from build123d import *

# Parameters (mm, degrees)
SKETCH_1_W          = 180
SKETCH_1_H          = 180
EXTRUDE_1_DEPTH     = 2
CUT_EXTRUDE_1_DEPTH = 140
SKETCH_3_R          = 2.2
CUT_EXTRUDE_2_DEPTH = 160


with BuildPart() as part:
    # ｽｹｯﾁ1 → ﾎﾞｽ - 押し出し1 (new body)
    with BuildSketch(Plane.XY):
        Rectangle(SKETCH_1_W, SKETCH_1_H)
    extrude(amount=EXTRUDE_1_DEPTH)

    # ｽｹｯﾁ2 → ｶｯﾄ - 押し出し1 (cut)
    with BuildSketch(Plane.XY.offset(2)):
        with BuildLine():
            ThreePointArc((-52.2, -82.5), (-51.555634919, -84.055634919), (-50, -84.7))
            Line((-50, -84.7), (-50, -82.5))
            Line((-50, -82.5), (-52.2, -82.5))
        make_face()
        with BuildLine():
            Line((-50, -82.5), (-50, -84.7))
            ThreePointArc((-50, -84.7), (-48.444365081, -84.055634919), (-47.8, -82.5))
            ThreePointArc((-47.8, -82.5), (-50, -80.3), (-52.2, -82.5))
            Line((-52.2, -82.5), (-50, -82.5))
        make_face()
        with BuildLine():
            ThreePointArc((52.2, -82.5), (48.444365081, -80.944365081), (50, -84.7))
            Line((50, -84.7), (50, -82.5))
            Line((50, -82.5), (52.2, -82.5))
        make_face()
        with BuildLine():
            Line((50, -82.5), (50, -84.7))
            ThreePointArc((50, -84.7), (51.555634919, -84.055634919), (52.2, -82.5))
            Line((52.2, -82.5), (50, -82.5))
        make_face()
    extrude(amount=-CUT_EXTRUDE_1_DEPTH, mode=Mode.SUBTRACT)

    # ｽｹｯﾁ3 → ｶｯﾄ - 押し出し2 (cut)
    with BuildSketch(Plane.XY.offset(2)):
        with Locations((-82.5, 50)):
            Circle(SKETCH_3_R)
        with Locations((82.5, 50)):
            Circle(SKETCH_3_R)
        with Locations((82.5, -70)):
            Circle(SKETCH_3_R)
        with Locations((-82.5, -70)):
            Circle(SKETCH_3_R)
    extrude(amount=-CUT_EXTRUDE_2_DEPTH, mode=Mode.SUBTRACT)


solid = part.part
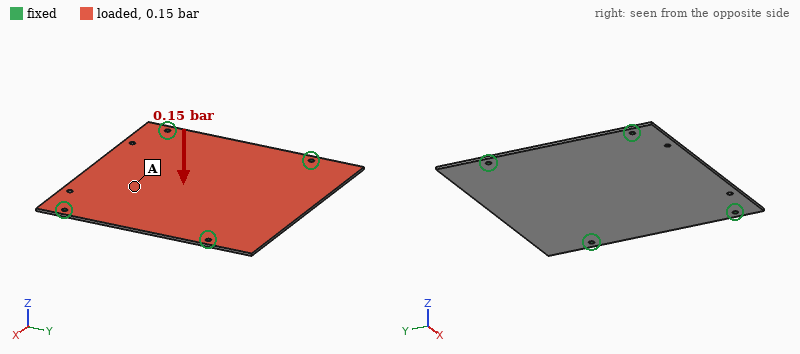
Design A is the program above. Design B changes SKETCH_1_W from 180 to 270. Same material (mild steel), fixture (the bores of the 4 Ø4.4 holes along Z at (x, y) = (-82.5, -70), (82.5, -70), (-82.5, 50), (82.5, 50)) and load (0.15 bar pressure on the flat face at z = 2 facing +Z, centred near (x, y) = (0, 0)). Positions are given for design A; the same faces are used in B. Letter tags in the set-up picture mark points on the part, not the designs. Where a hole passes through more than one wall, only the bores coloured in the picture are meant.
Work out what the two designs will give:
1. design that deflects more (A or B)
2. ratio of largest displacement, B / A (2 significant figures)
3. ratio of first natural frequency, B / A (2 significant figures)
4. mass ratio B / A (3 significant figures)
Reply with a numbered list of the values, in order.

1. A
2. 0.82
3. 1.00
4. 1.50
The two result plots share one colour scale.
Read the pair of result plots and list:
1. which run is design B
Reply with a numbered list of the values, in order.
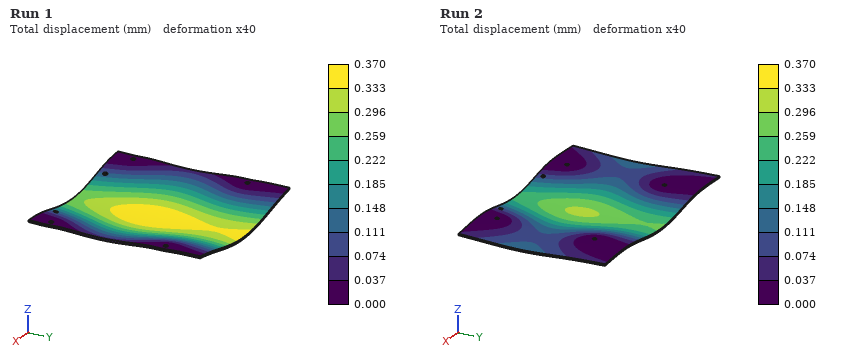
1. Run 2
